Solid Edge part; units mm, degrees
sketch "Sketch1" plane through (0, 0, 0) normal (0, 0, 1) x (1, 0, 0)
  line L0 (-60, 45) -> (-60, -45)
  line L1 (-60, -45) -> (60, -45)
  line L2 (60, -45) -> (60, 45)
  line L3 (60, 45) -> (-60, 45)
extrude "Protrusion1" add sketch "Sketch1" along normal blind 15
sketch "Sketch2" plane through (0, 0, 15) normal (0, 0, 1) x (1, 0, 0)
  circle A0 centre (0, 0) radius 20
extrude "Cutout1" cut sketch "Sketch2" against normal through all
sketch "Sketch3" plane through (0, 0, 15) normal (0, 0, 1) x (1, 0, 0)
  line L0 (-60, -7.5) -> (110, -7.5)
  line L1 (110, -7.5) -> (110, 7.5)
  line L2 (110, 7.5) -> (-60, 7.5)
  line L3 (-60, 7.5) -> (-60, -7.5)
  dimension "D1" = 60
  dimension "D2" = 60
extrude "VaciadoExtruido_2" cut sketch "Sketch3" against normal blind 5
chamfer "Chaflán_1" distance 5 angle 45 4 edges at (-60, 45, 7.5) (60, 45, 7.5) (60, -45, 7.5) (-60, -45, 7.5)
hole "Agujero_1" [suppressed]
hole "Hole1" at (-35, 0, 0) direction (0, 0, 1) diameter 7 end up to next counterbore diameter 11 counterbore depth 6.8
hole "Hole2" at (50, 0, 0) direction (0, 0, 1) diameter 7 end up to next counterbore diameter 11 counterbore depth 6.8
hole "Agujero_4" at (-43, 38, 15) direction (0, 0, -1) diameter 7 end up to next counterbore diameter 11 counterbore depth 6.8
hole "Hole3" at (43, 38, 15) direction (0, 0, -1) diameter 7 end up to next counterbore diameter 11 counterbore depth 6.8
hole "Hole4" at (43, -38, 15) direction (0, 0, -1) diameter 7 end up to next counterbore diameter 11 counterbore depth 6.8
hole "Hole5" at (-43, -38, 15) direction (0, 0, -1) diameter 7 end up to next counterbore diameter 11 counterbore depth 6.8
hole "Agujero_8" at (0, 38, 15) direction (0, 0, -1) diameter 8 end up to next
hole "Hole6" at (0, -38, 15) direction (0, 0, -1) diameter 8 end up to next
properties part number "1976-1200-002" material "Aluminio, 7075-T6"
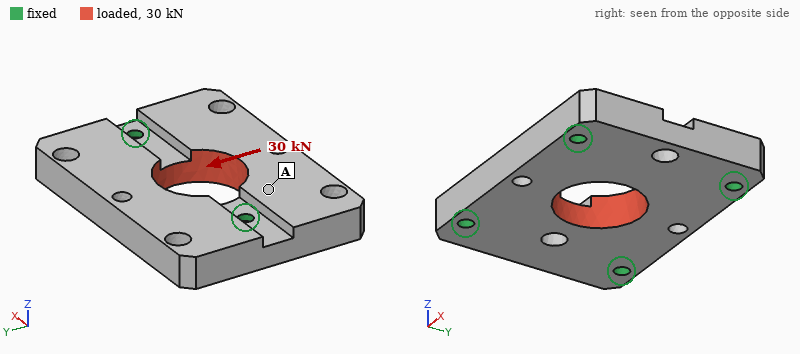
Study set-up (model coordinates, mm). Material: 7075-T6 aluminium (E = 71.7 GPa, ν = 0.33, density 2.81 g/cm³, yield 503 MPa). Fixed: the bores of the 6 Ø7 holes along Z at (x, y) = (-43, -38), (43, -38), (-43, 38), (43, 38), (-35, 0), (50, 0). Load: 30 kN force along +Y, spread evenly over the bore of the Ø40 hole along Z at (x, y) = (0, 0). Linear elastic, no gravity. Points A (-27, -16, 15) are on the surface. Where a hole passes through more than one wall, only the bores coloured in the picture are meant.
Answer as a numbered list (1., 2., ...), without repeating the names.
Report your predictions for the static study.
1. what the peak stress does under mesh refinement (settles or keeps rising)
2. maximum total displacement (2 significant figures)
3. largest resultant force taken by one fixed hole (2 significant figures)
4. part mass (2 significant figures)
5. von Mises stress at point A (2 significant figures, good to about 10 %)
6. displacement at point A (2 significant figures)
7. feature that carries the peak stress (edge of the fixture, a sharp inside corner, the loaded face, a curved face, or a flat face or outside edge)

1. keeps rising
2. 27 µm
3. 6.8 kN
4. 360 g
5. 19 MPa
6. 11 µm
7. edge of the fixture
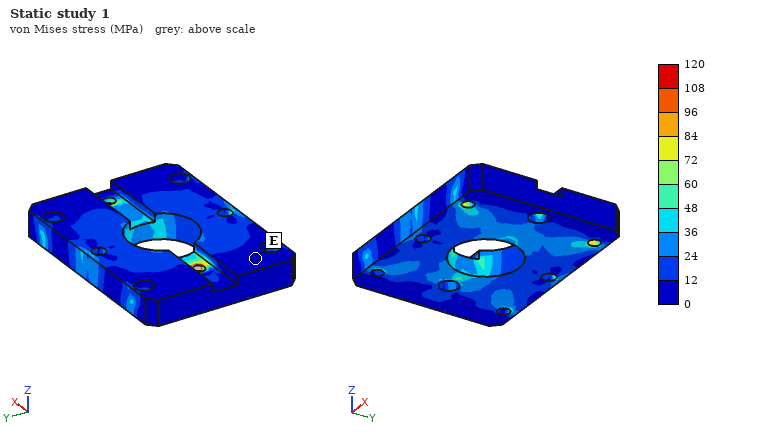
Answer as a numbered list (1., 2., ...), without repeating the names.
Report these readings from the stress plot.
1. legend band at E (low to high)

1. 0 to 12 MPa
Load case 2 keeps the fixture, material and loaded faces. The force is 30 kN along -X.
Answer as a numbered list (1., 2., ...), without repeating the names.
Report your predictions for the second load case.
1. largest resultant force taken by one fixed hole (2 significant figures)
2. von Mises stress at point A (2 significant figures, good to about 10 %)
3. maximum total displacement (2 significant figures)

1. 5.7 kN
2. 11 MPa
3. 12 µm
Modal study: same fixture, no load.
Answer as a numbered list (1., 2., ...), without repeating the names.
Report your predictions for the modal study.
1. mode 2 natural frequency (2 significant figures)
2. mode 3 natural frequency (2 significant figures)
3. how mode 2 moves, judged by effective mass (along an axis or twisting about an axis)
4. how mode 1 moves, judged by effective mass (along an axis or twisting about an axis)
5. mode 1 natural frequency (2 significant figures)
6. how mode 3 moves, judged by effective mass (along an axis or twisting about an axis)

1. 8000 Hz
2. 12 kHz
3. twisting about X
4. along Z
5. 6500 Hz
6. along Z
